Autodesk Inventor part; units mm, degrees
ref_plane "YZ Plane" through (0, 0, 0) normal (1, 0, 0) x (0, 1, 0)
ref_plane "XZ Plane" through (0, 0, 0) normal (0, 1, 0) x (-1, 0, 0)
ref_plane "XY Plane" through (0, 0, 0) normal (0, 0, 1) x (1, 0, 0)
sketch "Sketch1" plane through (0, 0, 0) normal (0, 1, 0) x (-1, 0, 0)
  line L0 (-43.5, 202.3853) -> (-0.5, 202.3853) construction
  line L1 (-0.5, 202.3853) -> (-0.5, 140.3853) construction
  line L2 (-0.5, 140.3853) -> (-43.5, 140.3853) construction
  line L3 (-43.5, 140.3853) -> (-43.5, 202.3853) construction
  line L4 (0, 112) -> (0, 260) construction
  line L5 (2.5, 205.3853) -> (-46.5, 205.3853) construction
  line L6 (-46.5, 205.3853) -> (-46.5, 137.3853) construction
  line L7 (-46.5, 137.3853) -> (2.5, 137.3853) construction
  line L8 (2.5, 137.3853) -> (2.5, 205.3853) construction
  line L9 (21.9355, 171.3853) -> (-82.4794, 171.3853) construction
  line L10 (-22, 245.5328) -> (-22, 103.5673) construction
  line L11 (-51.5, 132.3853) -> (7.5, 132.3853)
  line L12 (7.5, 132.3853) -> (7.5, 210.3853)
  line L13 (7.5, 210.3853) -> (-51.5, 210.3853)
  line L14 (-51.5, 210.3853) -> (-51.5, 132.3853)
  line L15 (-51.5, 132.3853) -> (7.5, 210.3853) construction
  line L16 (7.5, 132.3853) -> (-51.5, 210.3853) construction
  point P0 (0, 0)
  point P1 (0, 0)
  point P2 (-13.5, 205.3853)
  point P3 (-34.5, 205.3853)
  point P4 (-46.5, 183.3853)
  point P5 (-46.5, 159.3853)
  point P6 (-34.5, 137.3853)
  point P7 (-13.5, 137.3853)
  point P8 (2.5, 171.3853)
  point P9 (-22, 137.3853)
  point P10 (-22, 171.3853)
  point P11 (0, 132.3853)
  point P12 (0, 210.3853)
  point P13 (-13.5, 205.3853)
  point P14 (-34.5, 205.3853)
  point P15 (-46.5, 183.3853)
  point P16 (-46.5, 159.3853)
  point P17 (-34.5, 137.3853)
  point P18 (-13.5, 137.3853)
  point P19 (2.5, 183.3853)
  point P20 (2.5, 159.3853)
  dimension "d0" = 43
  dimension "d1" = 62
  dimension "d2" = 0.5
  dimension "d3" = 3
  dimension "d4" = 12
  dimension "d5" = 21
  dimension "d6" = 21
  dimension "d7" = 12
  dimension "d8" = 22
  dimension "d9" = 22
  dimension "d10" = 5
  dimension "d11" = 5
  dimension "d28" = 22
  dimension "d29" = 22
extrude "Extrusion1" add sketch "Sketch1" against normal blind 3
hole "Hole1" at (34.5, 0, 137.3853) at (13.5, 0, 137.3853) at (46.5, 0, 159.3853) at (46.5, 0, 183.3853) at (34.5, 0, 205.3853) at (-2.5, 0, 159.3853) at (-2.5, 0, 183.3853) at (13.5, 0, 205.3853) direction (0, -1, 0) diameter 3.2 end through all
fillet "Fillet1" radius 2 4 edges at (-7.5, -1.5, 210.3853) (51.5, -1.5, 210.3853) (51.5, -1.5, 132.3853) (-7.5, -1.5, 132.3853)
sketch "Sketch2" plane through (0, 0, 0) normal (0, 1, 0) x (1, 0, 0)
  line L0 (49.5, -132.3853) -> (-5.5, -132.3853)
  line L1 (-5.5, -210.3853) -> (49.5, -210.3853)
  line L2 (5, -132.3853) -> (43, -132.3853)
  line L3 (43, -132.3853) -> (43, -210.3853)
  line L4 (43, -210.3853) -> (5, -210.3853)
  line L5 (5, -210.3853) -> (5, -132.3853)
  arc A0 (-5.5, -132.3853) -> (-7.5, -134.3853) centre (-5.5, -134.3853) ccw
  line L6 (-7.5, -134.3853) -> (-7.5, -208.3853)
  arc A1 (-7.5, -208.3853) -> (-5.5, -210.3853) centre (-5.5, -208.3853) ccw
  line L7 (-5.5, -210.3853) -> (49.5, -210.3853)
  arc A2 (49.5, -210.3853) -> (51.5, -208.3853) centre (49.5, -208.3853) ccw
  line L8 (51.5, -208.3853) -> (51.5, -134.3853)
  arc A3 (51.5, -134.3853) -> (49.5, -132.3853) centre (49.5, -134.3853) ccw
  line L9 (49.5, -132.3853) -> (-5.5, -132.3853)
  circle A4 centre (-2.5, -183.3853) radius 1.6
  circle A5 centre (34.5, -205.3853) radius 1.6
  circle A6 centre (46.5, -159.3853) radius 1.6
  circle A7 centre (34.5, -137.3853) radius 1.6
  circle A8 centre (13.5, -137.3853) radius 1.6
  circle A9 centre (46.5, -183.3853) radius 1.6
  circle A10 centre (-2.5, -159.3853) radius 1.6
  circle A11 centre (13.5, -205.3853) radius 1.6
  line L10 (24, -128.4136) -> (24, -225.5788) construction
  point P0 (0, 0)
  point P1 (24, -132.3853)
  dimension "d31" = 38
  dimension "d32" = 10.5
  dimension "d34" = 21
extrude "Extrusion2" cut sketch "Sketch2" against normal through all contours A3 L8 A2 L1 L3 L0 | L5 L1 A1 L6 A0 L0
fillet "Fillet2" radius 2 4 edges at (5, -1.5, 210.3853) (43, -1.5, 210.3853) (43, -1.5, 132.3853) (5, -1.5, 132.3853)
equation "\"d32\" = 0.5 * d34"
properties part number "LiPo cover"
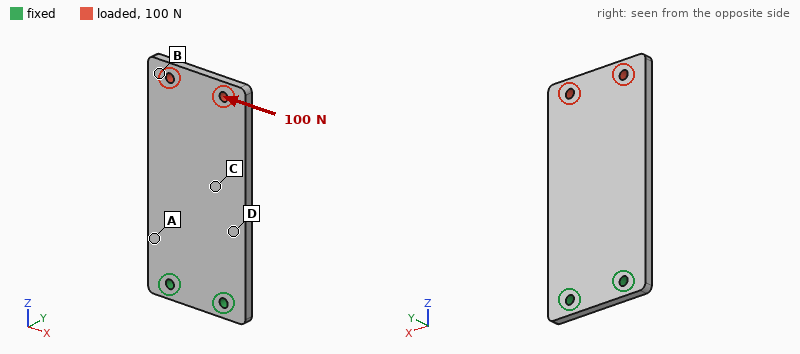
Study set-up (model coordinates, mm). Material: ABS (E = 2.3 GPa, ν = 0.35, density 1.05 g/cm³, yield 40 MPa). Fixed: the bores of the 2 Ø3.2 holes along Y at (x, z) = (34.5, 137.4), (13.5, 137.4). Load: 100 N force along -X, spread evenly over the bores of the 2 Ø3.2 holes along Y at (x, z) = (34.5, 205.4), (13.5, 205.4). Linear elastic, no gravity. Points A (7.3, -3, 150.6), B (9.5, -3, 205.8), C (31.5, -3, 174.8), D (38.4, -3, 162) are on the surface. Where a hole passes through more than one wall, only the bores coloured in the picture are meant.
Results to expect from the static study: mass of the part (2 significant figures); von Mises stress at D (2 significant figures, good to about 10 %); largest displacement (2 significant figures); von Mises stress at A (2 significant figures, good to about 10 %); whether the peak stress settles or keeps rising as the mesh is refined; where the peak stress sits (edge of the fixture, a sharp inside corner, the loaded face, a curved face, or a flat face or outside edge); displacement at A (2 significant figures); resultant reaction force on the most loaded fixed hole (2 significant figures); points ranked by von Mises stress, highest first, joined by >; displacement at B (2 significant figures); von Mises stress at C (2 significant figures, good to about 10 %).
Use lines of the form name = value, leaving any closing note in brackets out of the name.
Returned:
mass of the part = 9.2 g
von Mises stress at D = 4.6 MPa
largest displacement = 0.60 mm
von Mises stress at A = 6.1 MPa
whether the peak stress settles or keeps rising as the mesh is refined = keeps rising
where the peak stress sits = edge of the fixture
displacement at A = 0.100 mm
resultant reaction force on the most loaded fixed hole = 300 N
points ranked by von Mises stress, highest first, joined by > = A > D > C > B
displacement at B = 0.55 mm
von Mises stress at C = 2.5 MPa
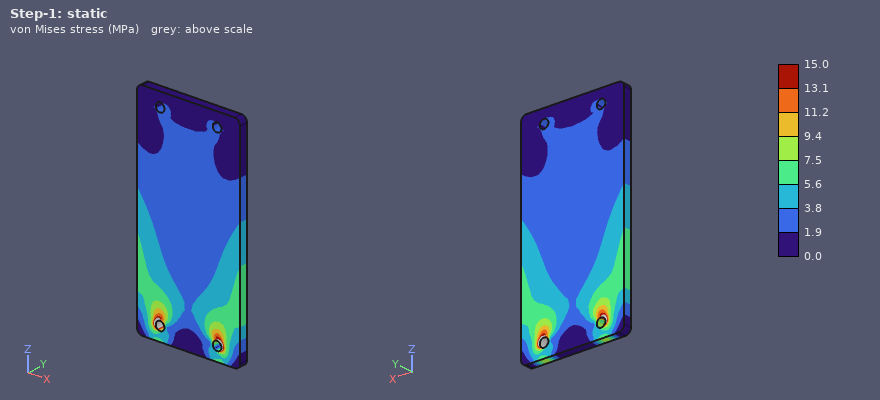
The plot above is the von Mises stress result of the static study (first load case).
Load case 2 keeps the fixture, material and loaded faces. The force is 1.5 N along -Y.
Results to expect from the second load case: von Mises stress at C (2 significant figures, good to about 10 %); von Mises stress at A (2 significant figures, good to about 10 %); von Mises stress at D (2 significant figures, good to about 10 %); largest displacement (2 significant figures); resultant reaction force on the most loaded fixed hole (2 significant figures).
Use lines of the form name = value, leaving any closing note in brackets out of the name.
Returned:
von Mises stress at C = 0.79 MPa
von Mises stress at A = 1.5 MPa
von Mises stress at D = 1.1 MPa
largest displacement = 0.88 mm
resultant reaction force on the most loaded fixed hole = 0.75 N
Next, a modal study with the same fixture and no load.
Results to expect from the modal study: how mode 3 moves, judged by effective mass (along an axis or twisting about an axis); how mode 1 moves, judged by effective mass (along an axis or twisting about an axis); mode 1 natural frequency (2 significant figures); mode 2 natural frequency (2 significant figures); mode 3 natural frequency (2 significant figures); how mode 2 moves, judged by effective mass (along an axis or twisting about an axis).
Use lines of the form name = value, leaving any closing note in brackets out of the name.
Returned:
how mode 3 moves, judged by effective mass = along Y
how mode 1 moves, judged by effective mass = along Y
mode 1 natural frequency = 140 Hz
mode 2 natural frequency = 550 Hz
mode 3 natural frequency = 840 Hz
how mode 2 moves, judged by effective mass = twisting about Z
